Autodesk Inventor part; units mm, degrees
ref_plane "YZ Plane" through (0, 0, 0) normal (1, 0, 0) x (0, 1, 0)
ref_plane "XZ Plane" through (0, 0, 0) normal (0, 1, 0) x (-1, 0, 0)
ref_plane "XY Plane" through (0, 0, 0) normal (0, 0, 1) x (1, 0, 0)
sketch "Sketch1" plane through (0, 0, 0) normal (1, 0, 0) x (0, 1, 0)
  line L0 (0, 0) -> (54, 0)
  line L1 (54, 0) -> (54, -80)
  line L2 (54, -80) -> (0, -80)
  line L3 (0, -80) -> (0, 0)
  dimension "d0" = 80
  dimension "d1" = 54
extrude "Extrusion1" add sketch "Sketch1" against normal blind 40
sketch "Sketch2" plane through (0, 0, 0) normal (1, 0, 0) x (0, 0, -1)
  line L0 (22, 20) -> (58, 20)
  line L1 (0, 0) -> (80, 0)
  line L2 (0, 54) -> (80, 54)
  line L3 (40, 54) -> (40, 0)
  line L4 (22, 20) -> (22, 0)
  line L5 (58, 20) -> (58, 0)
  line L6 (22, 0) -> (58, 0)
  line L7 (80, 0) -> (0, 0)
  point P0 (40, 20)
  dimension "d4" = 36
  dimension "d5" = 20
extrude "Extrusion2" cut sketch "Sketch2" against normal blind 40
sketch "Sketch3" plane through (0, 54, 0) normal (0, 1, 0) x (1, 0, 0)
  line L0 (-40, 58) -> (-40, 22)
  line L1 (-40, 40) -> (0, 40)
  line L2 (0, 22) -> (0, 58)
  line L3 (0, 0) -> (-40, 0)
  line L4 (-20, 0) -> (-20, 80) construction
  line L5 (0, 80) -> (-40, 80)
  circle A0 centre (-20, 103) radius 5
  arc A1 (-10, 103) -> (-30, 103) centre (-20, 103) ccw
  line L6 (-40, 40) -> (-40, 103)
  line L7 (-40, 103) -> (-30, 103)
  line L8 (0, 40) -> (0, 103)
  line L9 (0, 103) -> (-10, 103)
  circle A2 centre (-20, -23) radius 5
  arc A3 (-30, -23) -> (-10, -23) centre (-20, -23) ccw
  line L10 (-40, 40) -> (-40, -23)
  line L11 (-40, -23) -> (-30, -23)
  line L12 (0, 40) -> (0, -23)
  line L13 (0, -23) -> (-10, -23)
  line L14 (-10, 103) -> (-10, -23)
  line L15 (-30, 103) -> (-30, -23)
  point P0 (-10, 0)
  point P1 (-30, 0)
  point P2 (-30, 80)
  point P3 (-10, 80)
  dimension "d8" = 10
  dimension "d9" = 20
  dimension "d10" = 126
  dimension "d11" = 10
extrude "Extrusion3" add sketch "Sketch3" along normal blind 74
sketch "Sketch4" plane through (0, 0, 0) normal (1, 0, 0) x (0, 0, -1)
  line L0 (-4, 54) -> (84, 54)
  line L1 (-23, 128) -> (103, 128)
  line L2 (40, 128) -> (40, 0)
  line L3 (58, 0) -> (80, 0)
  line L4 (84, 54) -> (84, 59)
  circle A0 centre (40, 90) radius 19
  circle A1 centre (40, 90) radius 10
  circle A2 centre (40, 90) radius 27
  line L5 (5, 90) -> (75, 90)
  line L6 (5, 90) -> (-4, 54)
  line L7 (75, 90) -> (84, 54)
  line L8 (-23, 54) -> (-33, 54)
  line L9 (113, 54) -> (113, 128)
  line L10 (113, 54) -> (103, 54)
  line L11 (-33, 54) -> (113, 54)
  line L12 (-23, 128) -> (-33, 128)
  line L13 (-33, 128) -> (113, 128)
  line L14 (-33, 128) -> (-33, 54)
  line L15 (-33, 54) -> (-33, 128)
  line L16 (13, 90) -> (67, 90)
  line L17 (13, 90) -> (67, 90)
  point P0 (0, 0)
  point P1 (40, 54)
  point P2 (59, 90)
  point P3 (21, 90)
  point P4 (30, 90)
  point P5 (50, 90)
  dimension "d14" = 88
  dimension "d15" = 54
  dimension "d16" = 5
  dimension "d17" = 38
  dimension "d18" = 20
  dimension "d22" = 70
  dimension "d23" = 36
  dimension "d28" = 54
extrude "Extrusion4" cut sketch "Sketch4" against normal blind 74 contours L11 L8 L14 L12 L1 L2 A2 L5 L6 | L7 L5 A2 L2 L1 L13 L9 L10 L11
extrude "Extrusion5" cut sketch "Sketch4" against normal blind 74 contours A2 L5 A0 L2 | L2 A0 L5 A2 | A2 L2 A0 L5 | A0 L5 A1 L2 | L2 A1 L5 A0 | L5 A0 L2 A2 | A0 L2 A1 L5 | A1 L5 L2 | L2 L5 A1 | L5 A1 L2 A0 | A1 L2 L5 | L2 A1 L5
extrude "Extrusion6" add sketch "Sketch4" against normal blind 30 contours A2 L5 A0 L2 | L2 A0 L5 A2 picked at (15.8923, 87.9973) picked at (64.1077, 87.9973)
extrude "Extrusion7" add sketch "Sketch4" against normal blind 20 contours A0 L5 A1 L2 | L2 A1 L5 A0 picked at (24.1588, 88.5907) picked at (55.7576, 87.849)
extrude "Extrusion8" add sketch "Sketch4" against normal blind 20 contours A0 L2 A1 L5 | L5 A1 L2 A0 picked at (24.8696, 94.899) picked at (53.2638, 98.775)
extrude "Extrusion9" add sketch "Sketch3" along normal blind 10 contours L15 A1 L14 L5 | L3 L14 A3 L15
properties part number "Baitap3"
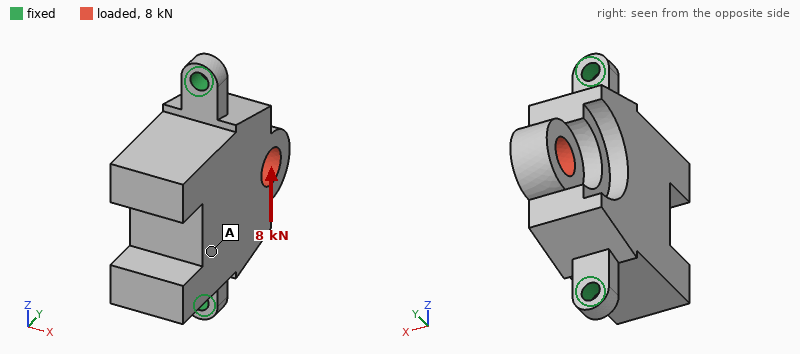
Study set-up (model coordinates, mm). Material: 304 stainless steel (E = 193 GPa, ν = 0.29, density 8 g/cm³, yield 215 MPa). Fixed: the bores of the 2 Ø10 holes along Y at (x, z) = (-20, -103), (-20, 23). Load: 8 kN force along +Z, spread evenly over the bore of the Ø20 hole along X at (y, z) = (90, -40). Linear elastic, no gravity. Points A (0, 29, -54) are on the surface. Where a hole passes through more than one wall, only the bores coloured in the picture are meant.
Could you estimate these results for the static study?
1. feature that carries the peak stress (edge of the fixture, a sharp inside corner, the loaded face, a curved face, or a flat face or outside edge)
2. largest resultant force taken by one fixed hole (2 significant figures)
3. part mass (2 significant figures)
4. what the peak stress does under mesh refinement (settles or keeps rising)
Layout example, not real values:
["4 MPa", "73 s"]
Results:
["edge of the fixture", "4.8 kN", "2.0 kg", "keeps rising"]
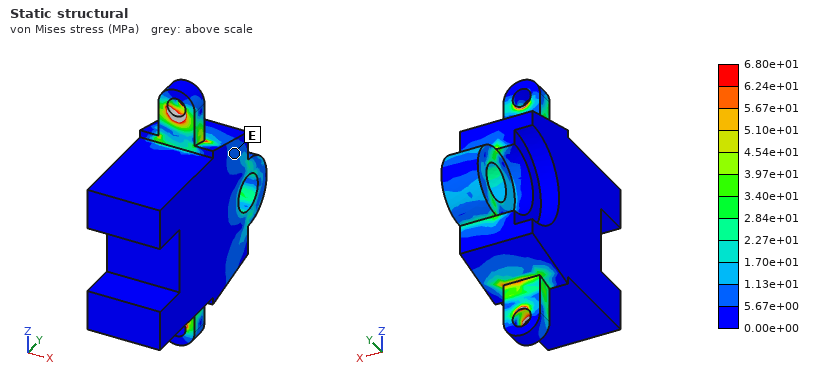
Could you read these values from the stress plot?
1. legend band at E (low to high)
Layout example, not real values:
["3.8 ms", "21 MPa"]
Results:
["5.67e+00 to 1.13e+01 MPa"]
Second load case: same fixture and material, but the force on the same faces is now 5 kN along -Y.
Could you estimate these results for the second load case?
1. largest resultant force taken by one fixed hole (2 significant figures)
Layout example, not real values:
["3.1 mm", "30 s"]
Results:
["2.5 kN"]
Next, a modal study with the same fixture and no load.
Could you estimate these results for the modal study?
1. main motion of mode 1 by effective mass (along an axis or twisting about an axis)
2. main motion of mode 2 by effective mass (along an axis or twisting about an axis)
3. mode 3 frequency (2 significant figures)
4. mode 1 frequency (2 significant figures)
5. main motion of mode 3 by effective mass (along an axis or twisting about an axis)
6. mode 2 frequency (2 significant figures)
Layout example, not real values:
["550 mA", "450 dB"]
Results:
["along X", "along Y", "3000 Hz", "760 Hz", "along X", "2400 Hz"]
